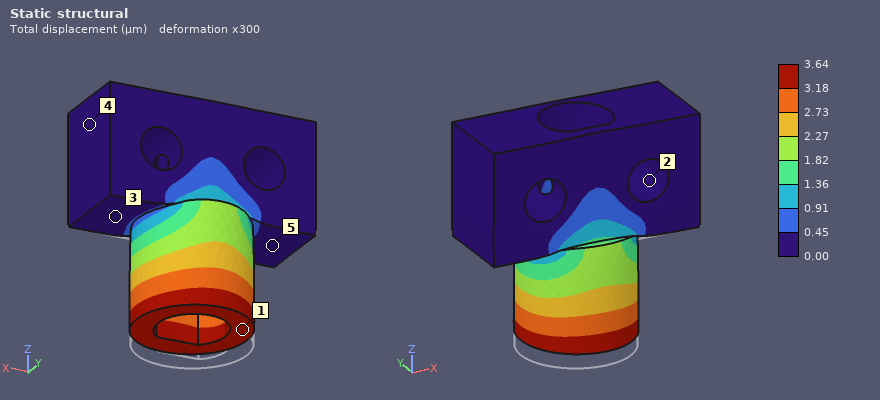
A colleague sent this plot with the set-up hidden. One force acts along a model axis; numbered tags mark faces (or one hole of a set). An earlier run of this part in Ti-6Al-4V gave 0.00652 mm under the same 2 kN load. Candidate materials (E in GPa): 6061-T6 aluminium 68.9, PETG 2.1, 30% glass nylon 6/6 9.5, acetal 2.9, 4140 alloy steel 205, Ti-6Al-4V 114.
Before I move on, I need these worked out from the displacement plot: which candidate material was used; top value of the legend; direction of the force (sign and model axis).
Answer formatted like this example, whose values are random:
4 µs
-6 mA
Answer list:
4140 alloy steel
3.64 µm
+Z
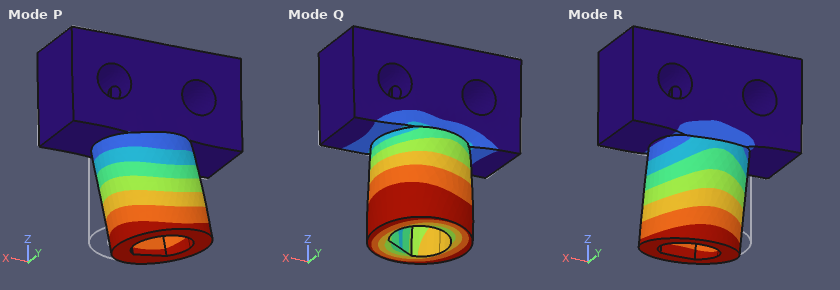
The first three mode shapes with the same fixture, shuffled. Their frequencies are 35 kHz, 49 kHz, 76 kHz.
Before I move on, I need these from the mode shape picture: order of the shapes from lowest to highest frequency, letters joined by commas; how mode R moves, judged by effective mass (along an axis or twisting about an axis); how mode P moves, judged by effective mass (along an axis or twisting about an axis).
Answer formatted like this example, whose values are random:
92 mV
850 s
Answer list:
R, P, Q
along Y
along X
